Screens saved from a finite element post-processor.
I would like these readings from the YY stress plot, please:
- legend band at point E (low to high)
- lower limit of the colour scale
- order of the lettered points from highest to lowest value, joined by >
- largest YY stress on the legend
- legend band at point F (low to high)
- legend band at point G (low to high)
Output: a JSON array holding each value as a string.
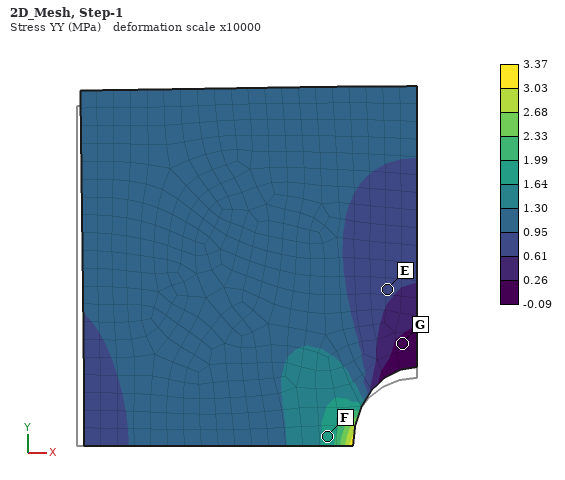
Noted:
["0.61 to 0.95 MPa", "-0.09 MPa", "F > E > G", "3.37 MPa", "1.64 to 1.99 MPa", "-0.09 to 0.26 MPa"]
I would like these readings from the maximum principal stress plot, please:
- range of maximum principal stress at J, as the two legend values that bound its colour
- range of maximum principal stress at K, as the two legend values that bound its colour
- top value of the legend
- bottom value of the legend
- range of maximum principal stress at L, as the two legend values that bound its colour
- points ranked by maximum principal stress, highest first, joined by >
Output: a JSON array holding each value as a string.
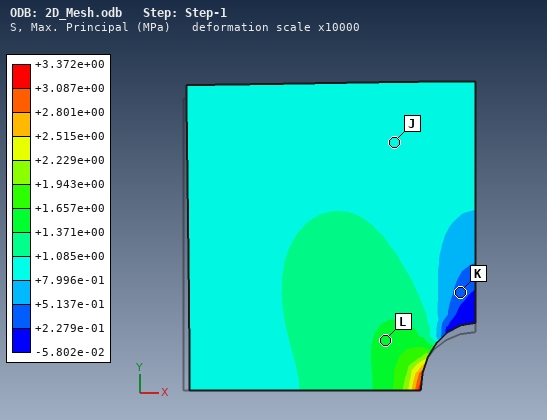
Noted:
["+7.996e-01 to +1.085e+00 MPa", "+2.279e-01 to +5.137e-01 MPa", "+3.372e+00 MPa", "-5.802e-02 MPa", "+1.371e+00 to +1.657e+00 MPa", "L > J > K"]
